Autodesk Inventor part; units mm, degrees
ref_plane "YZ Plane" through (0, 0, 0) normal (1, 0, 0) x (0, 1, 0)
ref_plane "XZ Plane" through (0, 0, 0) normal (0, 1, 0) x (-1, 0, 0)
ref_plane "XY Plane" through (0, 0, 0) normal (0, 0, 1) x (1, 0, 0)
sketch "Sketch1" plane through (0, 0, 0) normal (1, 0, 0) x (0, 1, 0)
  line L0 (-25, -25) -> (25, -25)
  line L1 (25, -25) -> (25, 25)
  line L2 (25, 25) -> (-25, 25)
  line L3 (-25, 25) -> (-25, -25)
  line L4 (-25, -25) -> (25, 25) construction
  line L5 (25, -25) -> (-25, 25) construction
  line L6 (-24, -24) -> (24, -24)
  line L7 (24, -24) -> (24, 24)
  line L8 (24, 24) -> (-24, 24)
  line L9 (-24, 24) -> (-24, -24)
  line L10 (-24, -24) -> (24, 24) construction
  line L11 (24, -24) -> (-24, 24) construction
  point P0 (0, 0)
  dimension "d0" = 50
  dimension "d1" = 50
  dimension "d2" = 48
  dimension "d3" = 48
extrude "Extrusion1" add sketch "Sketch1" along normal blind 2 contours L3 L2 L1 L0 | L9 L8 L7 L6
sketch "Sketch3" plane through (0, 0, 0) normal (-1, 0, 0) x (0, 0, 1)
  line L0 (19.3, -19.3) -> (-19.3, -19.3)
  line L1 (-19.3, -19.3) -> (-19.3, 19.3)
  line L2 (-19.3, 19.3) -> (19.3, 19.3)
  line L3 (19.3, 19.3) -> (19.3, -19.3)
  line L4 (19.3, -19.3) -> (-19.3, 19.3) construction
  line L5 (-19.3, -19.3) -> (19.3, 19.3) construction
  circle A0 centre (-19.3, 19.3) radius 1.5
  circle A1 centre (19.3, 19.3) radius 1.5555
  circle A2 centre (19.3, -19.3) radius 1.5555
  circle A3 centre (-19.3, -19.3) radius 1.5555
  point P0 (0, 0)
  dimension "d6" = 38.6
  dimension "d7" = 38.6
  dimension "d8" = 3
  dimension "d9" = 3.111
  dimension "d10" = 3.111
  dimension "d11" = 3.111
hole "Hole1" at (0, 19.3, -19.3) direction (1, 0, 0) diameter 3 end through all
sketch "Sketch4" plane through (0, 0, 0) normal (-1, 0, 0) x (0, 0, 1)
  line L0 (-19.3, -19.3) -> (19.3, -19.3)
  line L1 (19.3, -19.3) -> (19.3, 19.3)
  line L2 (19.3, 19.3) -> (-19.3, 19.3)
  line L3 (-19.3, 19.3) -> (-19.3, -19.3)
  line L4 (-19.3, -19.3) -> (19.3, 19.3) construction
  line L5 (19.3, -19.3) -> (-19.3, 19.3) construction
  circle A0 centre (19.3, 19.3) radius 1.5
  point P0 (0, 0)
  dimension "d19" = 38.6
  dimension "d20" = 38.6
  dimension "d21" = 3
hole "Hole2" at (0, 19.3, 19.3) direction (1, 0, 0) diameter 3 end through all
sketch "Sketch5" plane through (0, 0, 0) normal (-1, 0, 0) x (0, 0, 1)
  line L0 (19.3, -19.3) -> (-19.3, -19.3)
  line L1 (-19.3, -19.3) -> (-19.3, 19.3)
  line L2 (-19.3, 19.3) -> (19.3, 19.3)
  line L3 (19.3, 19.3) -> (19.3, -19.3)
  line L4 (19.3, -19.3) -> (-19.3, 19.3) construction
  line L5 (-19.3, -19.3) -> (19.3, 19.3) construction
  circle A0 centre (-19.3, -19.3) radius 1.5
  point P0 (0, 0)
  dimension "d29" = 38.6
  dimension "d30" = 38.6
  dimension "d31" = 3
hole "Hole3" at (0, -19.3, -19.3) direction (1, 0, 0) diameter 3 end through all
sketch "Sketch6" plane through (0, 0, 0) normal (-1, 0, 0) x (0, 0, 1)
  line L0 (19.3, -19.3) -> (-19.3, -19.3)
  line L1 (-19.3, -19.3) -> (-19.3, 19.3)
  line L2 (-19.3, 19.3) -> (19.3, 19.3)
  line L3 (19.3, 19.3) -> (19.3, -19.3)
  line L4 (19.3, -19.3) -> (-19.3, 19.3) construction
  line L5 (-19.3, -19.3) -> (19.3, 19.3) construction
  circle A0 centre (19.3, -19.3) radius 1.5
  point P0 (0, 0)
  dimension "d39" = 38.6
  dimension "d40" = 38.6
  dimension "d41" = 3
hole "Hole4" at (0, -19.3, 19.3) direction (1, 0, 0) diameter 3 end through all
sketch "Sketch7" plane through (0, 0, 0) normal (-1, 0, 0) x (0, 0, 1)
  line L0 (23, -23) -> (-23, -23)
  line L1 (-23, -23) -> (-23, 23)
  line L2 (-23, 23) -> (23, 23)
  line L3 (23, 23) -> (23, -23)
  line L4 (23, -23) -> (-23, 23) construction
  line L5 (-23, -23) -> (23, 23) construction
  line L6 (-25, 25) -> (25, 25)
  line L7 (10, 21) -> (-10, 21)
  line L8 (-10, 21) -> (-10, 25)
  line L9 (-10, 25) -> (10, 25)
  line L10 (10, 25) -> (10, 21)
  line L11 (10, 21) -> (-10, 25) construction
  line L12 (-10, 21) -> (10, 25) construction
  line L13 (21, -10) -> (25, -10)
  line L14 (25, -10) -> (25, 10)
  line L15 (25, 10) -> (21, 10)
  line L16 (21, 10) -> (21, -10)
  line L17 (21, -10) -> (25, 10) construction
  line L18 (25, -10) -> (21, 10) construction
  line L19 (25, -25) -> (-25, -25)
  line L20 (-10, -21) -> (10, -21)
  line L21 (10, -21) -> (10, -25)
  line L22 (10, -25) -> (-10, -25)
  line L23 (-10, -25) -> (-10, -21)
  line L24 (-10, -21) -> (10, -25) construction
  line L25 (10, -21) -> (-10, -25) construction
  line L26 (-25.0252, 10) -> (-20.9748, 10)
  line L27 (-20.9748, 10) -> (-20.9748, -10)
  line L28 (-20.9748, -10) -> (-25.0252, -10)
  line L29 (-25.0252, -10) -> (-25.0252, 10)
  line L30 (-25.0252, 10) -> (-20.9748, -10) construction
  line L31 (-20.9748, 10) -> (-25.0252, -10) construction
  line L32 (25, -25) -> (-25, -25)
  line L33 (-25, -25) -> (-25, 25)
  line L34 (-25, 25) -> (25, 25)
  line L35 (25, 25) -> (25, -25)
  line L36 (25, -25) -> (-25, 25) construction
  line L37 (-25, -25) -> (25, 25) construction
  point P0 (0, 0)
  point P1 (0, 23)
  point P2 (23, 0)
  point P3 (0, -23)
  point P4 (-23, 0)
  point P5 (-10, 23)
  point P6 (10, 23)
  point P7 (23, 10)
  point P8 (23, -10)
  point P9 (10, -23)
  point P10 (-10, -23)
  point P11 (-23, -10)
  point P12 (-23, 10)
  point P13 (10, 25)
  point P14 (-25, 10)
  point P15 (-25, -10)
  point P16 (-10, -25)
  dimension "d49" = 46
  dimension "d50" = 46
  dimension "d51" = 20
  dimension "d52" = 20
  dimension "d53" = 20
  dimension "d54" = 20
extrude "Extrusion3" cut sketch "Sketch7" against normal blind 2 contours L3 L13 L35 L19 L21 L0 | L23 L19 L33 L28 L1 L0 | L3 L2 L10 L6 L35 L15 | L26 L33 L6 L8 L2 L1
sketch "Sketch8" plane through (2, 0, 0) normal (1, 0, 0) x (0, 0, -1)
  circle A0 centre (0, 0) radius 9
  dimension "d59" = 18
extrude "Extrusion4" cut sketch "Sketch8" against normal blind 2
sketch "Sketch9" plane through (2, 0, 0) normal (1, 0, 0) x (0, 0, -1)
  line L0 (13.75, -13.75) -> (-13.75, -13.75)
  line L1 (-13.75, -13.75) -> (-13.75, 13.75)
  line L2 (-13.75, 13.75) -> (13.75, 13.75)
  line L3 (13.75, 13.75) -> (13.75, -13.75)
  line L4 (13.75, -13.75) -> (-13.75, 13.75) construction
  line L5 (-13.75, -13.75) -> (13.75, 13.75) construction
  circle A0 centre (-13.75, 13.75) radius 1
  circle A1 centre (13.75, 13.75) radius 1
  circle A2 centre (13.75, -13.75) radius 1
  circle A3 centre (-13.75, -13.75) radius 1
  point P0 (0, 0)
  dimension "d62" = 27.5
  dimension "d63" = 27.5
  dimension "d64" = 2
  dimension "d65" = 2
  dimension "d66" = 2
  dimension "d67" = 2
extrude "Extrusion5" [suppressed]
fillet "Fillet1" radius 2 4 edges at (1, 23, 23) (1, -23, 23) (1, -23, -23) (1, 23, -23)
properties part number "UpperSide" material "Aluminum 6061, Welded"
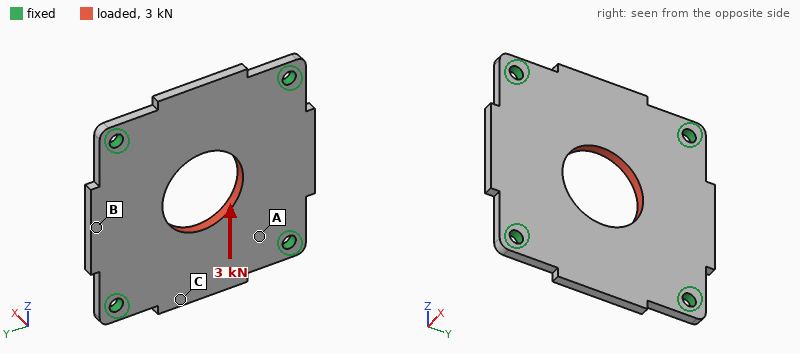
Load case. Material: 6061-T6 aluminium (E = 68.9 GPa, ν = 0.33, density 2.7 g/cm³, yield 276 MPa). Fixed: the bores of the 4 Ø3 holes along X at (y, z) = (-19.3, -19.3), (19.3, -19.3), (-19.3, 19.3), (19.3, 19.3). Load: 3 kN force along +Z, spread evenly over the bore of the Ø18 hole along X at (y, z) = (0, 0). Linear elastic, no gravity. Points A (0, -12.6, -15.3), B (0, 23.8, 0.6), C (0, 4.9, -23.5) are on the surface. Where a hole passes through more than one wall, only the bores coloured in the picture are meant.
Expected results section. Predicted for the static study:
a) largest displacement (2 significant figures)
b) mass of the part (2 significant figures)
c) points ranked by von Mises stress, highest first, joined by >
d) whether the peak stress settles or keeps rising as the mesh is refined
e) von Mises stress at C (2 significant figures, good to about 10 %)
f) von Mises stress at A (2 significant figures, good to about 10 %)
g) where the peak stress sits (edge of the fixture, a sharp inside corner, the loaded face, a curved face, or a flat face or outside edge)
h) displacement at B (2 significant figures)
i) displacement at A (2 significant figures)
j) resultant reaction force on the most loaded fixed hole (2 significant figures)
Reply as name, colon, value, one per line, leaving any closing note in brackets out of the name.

largest displacement: 15 µm
mass of the part: 11 g
points ranked by von Mises stress, highest first, joined by >: A > C > B
whether the peak stress settles or keeps rising as the mesh is refined: keeps rising
von Mises stress at C: 18 MPa
von Mises stress at A: 34 MPa
where the peak stress sits: edge of the fixture
displacement at B: 4.6 µm
displacement at A: 7.0 µm
resultant reaction force on the most loaded fixed hole: 810 N
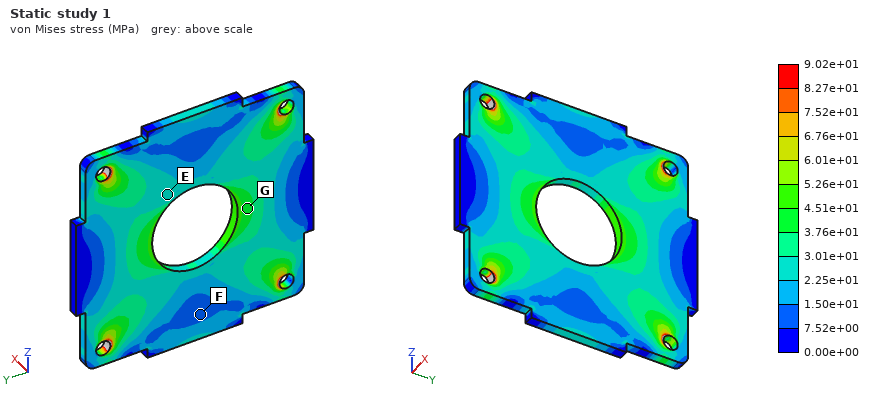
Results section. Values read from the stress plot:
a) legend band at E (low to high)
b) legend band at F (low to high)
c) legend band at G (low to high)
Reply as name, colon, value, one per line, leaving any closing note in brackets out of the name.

legend band at E: 2.25e+01 to 3.01e+01 MPa
legend band at F: 7.52e+00 to 1.50e+01 MPa
legend band at G: 3.76e+01 to 4.51e+01 MPa
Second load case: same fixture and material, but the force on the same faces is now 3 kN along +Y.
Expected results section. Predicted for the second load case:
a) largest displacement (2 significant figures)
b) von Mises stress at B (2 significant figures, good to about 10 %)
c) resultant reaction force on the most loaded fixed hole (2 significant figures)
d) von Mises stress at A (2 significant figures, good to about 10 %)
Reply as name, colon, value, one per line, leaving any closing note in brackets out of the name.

largest displacement: 15 µm
von Mises stress at B: 22 MPa
resultant reaction force on the most loaded fixed hole: 810 N
von Mises stress at A: 35 MPa
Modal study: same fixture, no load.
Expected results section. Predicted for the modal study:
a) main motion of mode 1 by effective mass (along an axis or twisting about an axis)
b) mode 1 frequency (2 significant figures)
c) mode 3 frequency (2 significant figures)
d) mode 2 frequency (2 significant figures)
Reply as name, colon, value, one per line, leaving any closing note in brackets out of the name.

main motion of mode 1 by effective mass: along X
mode 1 frequency: 5200 Hz
mode 3 frequency: 7300 Hz
mode 2 frequency: 7300 Hz
